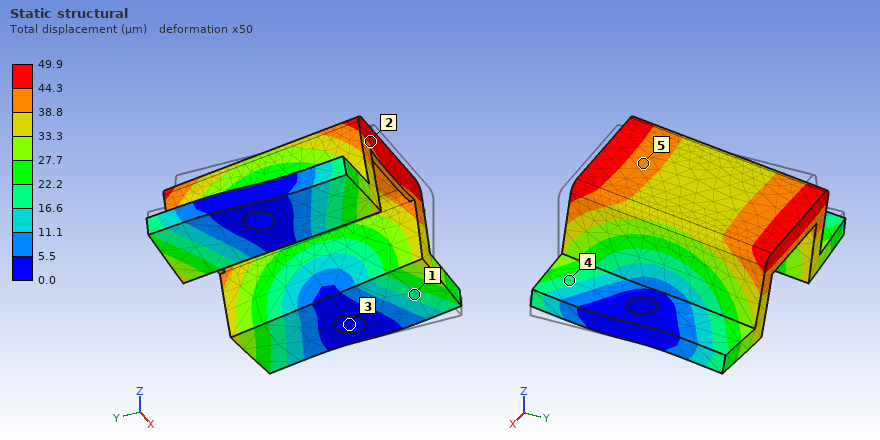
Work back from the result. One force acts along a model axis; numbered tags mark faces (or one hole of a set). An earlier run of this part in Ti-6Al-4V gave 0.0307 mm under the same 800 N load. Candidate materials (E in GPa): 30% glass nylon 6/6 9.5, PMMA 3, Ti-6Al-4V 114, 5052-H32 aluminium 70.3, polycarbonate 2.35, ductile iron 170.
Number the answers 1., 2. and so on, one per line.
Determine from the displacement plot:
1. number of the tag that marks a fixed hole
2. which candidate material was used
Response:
1. 3
2. 5052-H32 aluminium
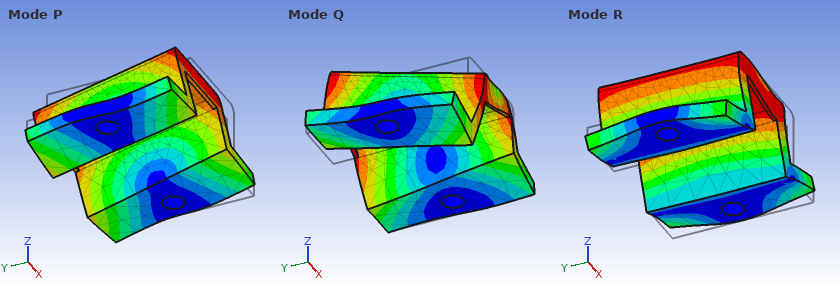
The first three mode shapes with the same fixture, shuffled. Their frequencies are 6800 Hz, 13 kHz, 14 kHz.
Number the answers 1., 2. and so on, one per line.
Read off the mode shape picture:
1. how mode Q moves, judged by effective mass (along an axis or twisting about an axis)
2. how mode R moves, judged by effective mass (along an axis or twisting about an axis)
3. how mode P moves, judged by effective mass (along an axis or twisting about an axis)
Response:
1. twisting about Z
2. along X
3. along Y
